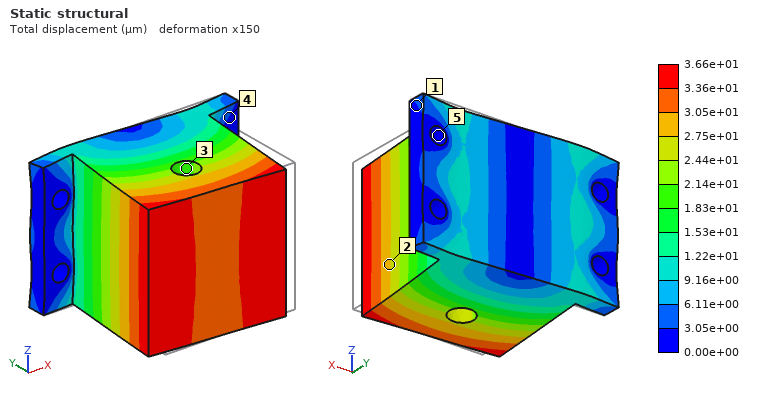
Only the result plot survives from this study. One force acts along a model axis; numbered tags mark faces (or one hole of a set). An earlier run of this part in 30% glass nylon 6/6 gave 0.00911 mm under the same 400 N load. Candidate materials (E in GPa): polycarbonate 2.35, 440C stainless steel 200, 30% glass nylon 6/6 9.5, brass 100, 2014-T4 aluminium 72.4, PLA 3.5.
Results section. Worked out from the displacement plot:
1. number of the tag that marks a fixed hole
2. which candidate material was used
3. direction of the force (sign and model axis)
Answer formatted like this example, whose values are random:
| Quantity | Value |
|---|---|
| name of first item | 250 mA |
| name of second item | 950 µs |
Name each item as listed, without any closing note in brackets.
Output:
| Quantity | Value |
|---|---|
| number of the tag that marks a fixed hole | 5 |
| which candidate material was used | polycarbonate |
| direction of the force | -X |
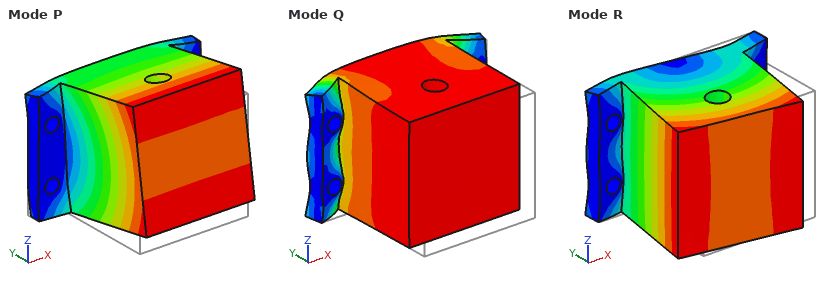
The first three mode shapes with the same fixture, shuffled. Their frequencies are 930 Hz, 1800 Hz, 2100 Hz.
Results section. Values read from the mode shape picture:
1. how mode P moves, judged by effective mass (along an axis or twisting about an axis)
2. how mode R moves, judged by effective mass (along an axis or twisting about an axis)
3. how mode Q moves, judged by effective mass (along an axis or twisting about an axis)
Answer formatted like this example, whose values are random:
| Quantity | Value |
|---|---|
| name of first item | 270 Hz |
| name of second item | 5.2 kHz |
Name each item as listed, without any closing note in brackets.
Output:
| Quantity | Value |
|---|---|
| how mode P moves, judged by effective mass | along Z |
| how mode R moves, judged by effective mass | along X |
| how mode Q moves, judged by effective mass | along Y |
